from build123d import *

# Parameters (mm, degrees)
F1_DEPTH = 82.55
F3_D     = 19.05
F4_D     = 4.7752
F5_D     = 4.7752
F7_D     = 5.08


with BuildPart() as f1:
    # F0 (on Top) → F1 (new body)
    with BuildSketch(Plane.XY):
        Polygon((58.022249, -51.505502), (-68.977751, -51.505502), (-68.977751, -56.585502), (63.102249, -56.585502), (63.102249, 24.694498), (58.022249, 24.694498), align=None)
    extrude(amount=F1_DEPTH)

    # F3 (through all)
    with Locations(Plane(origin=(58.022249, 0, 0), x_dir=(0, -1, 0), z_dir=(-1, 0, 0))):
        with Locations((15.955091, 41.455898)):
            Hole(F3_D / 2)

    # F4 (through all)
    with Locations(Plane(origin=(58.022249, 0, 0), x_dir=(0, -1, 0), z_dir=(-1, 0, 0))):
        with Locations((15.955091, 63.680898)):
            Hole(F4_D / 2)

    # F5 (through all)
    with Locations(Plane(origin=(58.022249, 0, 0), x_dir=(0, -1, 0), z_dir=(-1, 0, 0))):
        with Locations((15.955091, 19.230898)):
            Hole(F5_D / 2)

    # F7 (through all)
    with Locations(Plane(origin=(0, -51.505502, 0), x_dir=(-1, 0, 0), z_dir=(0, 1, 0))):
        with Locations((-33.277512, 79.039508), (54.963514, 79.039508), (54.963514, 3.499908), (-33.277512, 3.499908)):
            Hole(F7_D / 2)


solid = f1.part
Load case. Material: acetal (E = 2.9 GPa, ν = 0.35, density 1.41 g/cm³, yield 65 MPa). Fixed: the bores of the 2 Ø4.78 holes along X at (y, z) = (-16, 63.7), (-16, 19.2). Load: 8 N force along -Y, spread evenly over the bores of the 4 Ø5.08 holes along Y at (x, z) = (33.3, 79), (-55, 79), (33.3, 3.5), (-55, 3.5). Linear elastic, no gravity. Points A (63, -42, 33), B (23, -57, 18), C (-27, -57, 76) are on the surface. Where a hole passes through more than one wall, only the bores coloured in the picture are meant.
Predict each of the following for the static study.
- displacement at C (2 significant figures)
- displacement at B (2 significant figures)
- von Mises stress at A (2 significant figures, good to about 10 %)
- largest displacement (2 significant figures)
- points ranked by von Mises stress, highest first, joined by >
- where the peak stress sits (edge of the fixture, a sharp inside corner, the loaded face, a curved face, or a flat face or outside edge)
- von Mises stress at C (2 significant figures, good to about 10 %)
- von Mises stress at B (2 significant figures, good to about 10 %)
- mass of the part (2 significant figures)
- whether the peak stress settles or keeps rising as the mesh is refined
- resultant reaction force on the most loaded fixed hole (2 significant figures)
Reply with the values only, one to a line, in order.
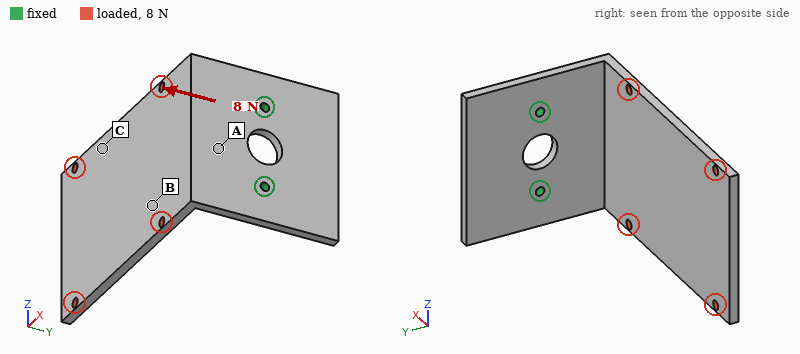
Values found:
1.3 mm
0.48 mm
1.4 MPa
2.0 mm
A > B > C
edge of the fixture
0.34 MPa
0.83 MPa
120 g
keeps rising
4.4 N
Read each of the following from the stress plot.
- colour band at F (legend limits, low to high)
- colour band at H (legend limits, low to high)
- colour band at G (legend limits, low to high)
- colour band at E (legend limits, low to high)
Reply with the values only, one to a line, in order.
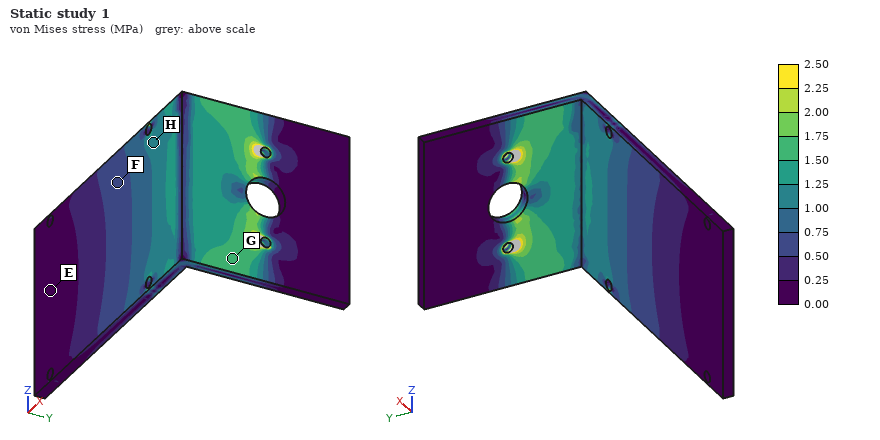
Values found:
0.50 to 0.75 MPa
1.00 to 1.25 MPa
1.50 to 1.75 MPa
0.00 to 0.25 MPa
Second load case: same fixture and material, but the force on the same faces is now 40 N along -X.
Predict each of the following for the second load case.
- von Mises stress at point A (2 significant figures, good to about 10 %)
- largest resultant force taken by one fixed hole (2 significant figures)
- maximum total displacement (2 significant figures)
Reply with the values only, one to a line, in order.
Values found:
1.2 MPa
20 N
1.7 mm
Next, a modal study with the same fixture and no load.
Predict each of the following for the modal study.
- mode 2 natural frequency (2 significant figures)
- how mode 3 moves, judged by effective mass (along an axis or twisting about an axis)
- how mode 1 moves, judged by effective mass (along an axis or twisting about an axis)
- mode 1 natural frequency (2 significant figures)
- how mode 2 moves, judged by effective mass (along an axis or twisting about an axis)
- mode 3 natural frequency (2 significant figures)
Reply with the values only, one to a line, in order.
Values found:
110 Hz
along X
along Y
47 Hz
along Z
230 Hz
